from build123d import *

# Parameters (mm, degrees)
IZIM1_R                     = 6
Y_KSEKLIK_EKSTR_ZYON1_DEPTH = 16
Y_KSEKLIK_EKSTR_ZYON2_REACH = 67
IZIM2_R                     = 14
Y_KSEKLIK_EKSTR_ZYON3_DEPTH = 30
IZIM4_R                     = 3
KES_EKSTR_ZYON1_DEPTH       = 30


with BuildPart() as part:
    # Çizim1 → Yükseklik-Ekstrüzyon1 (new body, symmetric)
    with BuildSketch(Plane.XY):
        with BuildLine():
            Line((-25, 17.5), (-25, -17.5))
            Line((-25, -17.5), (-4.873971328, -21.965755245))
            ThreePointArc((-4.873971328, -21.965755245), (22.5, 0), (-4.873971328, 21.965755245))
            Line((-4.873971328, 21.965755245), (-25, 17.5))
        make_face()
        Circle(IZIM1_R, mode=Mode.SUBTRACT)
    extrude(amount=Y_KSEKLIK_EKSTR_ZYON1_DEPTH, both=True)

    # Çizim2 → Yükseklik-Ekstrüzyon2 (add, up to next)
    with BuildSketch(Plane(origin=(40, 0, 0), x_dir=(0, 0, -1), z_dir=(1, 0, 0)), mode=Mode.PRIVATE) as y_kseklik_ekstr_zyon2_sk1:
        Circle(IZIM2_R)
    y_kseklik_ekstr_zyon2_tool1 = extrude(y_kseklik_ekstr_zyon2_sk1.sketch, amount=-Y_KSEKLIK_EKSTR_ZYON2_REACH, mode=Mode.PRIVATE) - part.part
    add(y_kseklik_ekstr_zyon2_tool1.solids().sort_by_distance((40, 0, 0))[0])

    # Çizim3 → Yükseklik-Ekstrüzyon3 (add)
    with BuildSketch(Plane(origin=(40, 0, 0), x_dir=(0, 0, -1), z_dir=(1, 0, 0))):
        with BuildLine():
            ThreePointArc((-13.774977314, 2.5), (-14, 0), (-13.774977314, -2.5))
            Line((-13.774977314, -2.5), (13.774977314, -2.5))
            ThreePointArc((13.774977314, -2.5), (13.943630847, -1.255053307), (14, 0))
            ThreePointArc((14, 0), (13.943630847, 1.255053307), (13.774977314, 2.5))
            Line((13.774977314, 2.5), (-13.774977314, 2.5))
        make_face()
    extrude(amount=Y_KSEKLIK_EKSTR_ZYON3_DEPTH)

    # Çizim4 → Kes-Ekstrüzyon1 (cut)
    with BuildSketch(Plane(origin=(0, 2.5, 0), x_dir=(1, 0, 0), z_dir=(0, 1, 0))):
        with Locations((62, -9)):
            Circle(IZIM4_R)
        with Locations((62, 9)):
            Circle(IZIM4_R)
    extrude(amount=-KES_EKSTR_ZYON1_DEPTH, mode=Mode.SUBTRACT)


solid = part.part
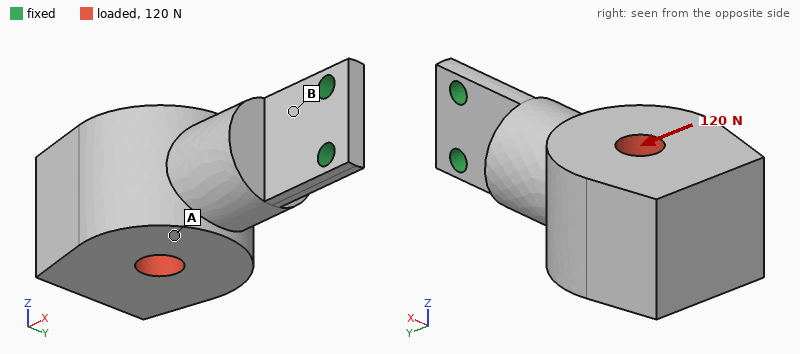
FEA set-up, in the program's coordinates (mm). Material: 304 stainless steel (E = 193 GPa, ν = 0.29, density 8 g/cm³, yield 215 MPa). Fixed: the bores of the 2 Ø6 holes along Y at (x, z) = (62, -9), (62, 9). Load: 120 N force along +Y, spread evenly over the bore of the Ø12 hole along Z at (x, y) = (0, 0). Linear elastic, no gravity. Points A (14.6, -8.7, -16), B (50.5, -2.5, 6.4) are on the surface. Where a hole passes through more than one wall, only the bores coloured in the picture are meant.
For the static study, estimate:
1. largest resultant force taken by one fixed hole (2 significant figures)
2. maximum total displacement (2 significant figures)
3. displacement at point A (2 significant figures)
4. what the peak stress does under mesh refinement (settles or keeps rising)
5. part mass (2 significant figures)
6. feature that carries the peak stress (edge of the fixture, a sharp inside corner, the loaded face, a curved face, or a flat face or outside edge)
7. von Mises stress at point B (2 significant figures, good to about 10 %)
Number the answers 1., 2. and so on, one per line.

1. 60 N
2. 0.18 mm
3. 0.083 mm
4. keeps rising
5. 560 g
6. edge of the fixture
7. 48 MPa
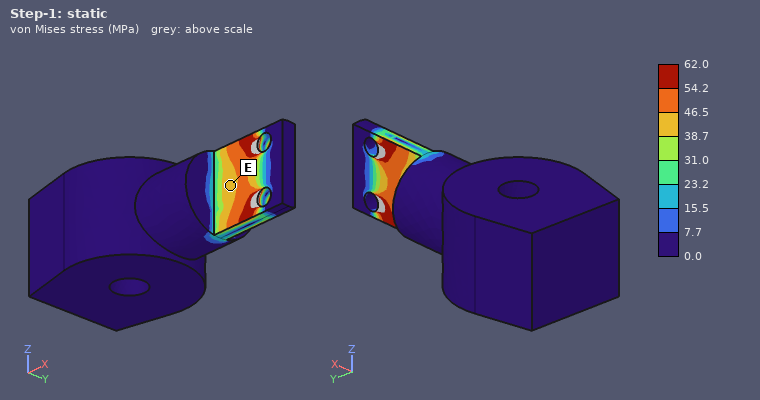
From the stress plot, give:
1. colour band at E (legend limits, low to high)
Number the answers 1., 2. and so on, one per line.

1. 38.7 to 46.5 MPa
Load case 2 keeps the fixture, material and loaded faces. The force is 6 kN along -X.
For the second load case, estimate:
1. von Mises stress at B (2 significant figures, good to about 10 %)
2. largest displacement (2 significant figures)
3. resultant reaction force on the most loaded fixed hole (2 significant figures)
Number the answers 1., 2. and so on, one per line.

1. 45 MPa
2. 7.7 µm
3. 3.0 kN
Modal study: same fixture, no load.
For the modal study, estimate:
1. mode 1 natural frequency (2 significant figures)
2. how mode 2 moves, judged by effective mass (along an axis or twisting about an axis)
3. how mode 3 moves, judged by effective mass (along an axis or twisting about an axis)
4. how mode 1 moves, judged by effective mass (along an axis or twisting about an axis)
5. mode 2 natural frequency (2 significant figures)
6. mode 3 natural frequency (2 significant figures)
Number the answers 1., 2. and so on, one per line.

1. 220 Hz
2. along Z
3. twisting about X
4. along Y
5. 1100 Hz
6. 1300 Hz
